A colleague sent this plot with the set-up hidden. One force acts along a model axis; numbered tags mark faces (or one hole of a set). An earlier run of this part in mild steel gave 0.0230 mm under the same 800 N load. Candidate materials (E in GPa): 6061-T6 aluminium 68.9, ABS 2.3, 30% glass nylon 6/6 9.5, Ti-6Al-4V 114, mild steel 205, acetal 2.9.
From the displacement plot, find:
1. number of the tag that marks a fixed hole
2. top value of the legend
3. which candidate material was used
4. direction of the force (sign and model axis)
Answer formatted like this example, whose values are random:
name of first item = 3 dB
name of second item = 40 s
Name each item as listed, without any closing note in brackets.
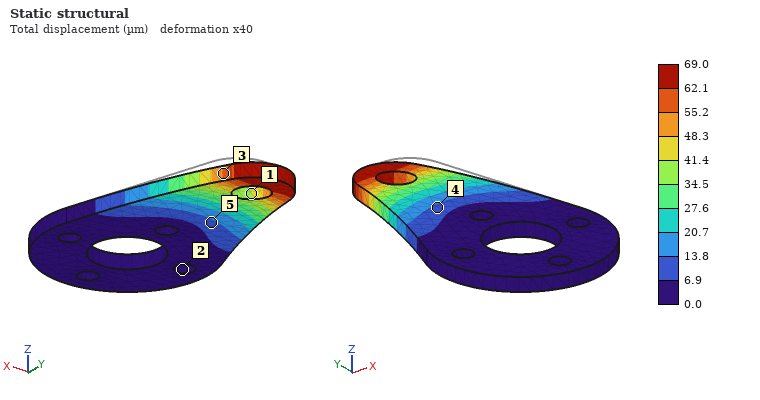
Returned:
number of the tag that marks a fixed hole = 2
top value of the legend = 69.0 µm
which candidate material was used = 6061-T6 aluminium
direction of the force = -X
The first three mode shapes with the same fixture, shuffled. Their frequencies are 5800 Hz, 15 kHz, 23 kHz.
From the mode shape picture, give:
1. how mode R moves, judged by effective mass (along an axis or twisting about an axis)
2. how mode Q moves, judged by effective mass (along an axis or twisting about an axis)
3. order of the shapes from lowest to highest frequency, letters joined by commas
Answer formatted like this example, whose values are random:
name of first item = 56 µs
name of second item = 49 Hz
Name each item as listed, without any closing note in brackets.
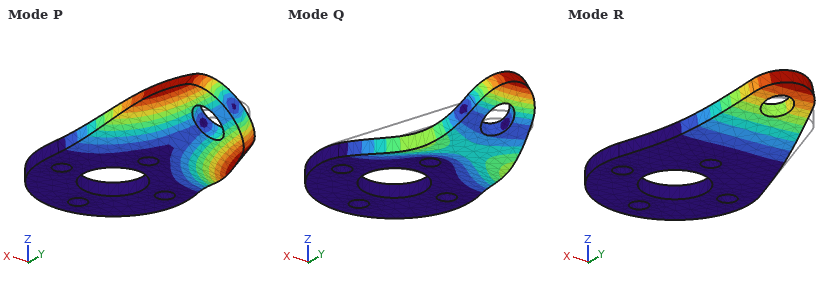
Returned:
how mode R moves, judged by effective mass = along Z
how mode Q moves, judged by effective mass = along Z
order of the shapes from lowest to highest frequency, letters joined by commas = R, P, Q
